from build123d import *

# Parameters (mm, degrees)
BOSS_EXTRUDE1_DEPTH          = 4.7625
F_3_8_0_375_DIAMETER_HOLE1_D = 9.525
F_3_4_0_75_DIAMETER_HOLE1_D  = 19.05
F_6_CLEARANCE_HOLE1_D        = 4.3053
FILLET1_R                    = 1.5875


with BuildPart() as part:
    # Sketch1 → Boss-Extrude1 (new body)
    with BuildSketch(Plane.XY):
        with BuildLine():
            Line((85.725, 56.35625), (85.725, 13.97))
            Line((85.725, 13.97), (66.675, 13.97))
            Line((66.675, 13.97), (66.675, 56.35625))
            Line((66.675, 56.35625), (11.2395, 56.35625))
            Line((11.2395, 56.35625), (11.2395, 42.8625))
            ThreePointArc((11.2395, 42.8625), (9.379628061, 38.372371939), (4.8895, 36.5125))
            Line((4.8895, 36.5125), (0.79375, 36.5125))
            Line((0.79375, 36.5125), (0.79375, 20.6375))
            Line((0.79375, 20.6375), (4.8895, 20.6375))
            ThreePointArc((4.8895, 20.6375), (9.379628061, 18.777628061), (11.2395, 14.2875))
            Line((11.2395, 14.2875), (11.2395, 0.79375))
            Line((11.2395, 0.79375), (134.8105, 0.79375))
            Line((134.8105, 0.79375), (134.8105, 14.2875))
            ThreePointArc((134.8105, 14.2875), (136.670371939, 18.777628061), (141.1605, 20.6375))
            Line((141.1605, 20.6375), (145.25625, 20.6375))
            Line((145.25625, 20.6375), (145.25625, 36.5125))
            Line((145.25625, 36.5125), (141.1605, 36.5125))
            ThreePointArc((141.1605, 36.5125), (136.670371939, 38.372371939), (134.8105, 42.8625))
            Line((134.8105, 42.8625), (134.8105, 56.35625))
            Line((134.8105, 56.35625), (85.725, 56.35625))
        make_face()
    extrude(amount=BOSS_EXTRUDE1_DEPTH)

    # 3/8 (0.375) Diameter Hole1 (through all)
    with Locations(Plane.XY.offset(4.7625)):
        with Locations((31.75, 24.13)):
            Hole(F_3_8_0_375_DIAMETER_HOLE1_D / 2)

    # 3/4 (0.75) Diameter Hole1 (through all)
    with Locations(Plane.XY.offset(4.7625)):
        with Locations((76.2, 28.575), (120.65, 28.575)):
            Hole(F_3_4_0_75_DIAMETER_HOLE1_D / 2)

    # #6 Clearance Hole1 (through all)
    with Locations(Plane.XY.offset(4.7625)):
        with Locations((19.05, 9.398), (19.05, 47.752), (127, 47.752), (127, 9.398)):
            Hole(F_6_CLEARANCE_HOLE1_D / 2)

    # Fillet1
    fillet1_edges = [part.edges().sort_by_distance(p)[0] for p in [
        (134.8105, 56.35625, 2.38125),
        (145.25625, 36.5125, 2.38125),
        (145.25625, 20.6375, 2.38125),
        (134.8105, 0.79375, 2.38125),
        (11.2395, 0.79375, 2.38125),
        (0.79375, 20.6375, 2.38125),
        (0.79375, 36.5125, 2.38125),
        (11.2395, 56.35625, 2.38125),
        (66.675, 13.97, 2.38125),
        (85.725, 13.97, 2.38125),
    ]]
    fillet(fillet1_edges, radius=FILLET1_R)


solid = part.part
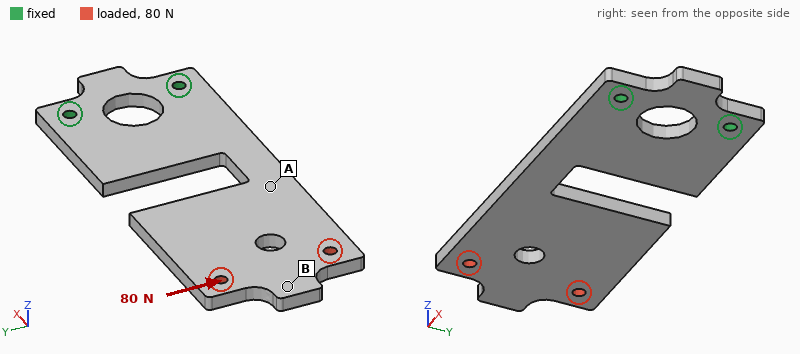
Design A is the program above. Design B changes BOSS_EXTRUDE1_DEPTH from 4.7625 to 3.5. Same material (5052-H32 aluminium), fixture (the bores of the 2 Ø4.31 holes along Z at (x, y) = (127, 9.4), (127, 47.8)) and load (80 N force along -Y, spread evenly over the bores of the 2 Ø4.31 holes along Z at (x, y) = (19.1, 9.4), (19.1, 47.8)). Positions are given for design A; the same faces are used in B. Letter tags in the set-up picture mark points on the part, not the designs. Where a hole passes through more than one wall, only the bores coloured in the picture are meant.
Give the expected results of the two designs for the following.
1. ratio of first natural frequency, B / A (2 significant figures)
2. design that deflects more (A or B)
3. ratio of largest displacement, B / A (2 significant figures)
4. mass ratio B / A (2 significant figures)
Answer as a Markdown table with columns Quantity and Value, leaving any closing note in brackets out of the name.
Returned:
| Quantity | Value |
|---|---|
| ratio of first natural frequency, B / A | 0.74 |
| design that deflects more | B |
| ratio of largest displacement, B / A | 1.4 |
| mass ratio B / A | 0.73 |
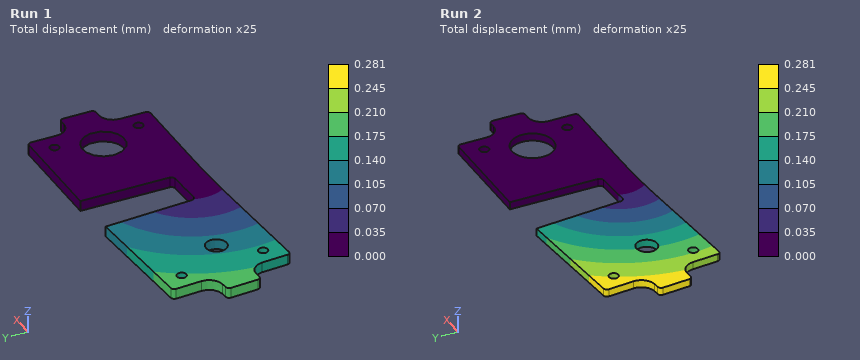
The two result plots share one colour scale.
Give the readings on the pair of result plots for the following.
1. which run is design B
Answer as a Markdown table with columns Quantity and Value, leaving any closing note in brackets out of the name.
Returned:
| Quantity | Value |
|---|---|
| which run is design B | Run 2 |
